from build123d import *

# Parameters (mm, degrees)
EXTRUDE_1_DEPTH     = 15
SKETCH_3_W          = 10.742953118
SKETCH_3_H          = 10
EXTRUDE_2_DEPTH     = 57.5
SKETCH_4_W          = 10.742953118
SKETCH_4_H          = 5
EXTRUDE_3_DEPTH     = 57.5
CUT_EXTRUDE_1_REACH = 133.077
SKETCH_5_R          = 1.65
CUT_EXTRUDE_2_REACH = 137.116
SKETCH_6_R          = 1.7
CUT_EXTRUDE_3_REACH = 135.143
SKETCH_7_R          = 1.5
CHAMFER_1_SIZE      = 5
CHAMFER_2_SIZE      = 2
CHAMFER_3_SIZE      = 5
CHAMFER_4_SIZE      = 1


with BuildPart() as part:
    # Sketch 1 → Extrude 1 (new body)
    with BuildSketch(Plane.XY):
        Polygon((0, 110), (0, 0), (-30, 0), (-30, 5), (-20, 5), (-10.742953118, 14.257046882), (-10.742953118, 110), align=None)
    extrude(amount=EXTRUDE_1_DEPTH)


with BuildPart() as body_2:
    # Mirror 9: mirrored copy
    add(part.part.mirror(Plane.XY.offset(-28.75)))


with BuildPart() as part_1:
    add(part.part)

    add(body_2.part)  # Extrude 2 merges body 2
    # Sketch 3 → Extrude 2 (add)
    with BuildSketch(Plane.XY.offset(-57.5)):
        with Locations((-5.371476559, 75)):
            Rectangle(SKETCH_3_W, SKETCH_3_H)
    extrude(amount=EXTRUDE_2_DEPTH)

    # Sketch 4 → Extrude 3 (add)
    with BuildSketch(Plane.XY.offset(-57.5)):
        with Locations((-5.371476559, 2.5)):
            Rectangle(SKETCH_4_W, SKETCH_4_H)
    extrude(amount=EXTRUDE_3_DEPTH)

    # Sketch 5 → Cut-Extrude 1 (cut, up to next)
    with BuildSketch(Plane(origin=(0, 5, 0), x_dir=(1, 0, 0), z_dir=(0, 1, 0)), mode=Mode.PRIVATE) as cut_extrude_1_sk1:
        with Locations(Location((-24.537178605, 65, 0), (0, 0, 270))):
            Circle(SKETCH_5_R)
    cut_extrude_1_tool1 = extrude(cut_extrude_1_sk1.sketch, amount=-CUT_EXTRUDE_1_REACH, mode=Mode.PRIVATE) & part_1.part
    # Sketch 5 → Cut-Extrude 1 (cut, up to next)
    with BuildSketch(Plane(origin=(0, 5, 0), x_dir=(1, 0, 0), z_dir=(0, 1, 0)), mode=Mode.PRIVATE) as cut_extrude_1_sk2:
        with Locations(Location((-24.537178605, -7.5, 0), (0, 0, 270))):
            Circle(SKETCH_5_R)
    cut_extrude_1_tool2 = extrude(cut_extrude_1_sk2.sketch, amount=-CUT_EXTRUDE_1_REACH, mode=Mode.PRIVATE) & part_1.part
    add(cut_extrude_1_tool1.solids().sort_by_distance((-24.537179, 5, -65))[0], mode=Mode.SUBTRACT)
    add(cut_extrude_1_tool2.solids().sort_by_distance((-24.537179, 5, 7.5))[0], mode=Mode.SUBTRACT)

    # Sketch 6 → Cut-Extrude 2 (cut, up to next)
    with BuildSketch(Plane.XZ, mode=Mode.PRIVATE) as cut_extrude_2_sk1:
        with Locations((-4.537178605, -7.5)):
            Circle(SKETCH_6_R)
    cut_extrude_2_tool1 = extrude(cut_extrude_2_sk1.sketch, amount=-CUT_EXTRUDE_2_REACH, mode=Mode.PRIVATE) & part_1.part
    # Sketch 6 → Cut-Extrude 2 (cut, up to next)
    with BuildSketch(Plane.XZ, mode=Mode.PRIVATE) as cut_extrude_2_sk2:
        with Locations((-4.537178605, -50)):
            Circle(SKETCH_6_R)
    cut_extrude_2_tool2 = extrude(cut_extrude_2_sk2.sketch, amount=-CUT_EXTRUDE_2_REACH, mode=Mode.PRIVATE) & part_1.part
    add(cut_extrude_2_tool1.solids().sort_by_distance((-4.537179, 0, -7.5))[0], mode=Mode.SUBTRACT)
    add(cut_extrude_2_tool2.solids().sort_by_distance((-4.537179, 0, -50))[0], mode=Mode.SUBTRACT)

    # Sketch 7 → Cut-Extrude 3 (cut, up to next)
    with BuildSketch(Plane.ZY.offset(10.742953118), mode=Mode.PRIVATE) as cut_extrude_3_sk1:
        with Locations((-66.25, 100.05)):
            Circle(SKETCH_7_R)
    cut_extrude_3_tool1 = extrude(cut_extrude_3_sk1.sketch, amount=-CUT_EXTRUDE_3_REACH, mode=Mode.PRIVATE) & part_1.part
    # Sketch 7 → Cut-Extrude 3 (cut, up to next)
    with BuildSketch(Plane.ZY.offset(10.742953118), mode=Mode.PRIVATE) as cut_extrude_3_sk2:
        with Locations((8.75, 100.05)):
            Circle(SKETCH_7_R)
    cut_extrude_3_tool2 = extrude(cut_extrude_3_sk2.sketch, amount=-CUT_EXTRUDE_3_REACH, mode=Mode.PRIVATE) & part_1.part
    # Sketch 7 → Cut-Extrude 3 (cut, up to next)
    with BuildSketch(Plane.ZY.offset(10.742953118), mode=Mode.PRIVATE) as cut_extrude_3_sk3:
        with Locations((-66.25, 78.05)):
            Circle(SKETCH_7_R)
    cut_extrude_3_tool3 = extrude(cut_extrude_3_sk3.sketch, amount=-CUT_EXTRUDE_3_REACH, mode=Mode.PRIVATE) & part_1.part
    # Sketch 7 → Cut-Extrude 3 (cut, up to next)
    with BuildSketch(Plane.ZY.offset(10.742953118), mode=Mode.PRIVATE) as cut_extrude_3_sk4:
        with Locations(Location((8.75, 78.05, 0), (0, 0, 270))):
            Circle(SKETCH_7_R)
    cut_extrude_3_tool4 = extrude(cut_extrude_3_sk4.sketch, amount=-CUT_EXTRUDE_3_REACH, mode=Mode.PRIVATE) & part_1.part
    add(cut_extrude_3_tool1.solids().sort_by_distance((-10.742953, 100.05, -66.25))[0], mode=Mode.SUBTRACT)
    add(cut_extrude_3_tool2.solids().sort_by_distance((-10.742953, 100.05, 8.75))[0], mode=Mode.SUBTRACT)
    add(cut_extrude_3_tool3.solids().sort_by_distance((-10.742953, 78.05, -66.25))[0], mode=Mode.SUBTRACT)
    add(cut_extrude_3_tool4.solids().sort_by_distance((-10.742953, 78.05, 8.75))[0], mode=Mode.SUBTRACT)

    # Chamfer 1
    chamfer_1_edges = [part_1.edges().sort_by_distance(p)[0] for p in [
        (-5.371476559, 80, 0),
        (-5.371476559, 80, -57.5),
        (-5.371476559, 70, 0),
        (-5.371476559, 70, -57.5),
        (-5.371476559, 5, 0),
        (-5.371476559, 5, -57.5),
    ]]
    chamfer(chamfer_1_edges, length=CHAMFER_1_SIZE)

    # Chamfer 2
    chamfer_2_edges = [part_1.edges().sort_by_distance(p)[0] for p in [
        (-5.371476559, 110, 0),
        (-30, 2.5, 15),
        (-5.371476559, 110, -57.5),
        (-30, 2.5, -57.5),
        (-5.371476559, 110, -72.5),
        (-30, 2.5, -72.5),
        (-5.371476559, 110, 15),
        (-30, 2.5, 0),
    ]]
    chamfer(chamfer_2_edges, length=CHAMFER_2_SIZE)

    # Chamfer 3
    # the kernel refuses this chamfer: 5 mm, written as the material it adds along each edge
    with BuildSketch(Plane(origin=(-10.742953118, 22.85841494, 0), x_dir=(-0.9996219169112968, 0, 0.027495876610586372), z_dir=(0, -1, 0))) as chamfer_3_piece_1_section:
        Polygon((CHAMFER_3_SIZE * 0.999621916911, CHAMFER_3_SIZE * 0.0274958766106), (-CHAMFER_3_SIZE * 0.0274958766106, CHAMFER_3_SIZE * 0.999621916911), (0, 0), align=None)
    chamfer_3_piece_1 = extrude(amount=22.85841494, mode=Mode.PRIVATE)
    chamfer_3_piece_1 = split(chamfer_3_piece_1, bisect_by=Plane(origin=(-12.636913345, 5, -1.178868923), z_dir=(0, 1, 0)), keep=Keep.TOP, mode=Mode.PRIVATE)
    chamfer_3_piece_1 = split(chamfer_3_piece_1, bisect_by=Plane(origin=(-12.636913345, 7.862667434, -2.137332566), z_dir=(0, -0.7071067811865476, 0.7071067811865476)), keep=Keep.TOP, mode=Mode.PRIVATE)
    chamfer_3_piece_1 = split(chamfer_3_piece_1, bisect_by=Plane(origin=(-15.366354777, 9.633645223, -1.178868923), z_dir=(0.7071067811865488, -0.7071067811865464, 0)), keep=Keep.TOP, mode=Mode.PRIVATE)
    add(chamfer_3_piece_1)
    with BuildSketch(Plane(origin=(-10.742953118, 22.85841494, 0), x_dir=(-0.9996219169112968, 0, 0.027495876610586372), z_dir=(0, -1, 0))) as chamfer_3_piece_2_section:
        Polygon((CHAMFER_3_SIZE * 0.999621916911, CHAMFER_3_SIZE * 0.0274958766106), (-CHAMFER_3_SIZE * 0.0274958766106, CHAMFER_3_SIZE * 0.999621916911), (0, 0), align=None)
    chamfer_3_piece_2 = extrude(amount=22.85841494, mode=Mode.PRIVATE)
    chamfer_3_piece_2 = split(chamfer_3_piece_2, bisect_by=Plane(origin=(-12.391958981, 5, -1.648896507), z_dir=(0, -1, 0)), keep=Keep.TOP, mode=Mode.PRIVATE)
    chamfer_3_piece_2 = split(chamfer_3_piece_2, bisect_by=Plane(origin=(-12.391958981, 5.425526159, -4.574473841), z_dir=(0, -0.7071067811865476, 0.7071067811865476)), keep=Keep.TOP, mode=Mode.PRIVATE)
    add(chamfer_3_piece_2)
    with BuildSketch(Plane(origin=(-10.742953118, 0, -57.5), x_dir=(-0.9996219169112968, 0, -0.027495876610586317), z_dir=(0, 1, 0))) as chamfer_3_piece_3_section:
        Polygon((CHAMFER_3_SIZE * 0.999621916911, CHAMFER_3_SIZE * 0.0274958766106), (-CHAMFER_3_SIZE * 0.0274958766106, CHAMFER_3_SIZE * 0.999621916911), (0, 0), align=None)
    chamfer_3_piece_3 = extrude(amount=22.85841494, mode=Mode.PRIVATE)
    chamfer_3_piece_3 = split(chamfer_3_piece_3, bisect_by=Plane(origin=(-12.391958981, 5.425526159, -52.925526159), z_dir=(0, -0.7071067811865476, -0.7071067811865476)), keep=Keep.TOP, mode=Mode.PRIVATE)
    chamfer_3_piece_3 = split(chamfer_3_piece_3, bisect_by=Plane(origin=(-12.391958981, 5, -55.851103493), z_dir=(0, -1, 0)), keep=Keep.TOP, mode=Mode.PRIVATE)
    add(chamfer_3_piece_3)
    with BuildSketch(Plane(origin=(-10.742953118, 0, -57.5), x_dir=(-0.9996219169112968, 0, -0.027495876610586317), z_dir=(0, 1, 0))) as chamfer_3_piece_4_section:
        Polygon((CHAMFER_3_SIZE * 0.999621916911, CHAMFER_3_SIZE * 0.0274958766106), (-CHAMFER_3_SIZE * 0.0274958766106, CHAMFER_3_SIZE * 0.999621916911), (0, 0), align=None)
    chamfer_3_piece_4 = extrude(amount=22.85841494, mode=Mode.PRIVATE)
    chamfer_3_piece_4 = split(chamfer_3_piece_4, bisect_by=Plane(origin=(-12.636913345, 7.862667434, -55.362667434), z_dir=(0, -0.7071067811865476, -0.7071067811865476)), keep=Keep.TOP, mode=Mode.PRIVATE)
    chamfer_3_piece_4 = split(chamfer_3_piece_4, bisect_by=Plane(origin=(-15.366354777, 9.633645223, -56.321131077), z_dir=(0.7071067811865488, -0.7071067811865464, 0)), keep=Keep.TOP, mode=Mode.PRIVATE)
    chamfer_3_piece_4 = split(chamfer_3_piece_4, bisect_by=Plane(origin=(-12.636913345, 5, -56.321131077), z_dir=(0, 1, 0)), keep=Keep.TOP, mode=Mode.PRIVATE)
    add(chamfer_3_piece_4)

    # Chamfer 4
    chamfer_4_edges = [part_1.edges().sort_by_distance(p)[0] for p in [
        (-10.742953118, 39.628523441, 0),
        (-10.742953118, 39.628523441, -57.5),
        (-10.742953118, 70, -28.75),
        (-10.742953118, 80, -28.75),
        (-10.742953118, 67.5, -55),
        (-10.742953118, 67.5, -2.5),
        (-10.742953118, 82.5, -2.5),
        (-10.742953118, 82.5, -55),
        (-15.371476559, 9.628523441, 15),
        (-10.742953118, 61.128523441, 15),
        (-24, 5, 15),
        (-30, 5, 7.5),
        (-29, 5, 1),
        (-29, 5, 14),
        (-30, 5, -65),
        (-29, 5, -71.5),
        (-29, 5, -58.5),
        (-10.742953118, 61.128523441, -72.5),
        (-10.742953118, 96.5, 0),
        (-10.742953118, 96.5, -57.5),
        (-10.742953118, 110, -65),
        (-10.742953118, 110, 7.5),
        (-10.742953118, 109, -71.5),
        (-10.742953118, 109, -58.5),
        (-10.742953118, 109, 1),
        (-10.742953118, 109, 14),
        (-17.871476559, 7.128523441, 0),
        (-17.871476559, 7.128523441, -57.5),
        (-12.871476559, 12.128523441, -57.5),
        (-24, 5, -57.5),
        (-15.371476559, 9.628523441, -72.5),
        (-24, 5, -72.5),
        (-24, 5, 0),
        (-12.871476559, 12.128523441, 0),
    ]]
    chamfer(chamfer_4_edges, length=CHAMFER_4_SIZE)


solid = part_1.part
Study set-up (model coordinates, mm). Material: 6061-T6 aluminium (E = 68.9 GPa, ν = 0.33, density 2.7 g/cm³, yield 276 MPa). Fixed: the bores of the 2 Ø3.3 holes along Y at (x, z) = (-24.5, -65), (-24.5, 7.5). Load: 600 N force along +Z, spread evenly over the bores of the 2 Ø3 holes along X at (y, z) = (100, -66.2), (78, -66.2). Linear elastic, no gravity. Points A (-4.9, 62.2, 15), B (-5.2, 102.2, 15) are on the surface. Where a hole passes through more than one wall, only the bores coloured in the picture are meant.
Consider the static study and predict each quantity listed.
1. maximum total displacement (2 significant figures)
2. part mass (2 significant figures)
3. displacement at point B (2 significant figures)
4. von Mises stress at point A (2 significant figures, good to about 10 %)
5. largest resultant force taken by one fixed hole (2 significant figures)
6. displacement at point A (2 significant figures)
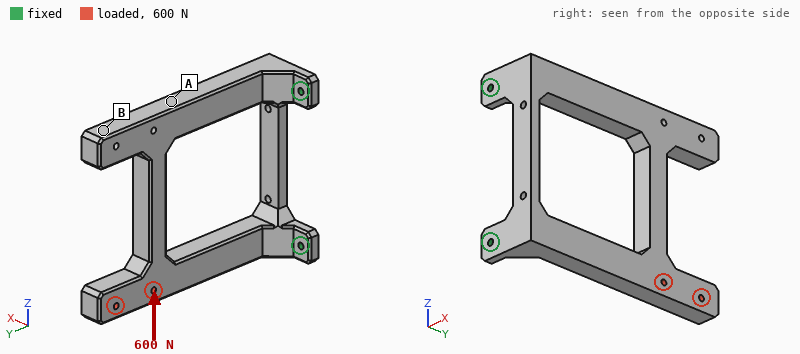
0.39 mm
130 g
0.33 mm
27 MPa
640 N
0.24 mm
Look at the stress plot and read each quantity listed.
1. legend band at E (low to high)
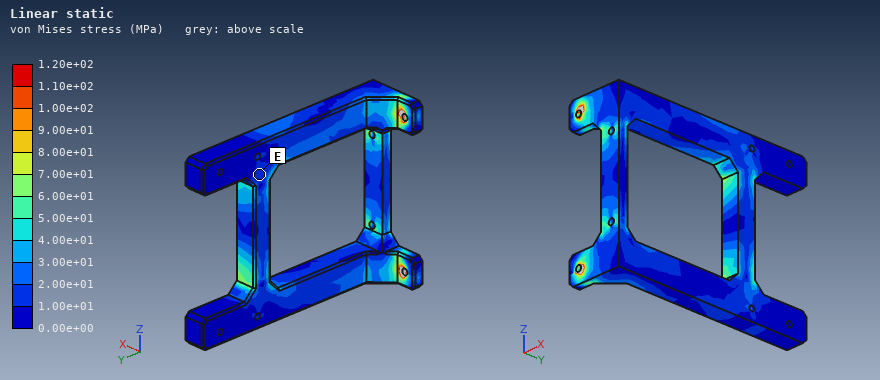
1.00e+01 to 2.00e+01 MPa
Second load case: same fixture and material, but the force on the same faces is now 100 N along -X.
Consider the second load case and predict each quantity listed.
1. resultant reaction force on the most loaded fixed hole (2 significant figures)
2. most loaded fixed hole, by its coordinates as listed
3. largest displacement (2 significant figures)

90 N
(-24.5, -65)
0.55 mm
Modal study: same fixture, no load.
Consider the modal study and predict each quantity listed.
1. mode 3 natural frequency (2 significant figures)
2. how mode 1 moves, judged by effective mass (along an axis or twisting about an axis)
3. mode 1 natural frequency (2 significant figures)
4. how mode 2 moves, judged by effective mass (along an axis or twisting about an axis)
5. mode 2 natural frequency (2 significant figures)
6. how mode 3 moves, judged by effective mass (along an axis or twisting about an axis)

1100 Hz
along X
340 Hz
along Z
830 Hz
along Z
